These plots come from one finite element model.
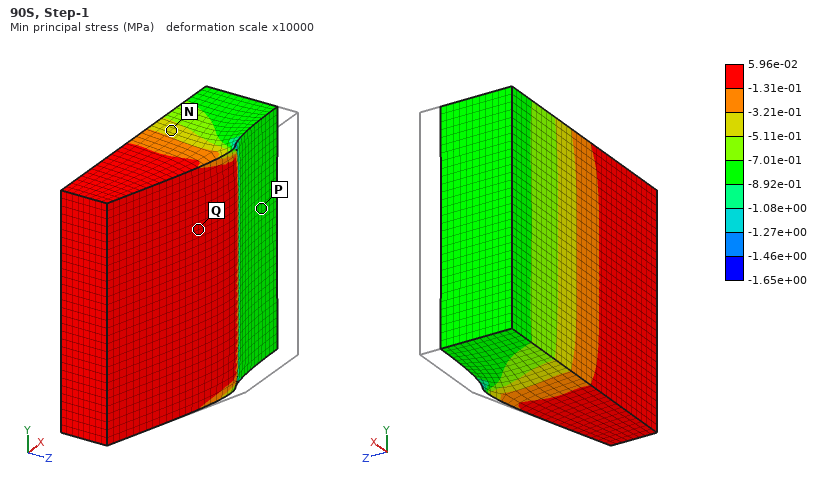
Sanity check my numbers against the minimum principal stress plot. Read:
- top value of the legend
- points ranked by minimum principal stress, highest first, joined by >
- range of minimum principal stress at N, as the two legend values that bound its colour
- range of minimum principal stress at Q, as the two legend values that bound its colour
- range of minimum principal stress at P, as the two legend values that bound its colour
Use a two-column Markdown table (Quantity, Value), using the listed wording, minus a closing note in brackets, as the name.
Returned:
| Quantity | Value |
|---|---|
| top value of the legend | 5.96e-02 MPa |
| points ranked by minimum principal stress, highest first, joined by > | Q > N > P |
| range of minimum principal stress at N, as the two legend values that bound its colour | -5.11e-01 to -3.21e-01 MPa |
| range of minimum principal stress at Q, as the two legend values that bound its colour | -1.31e-01 to 5.96e-02 MPa |
| range of minimum principal stress at P, as the two legend values that bound its colour | -8.92e-01 to -7.01e-01 MPa |
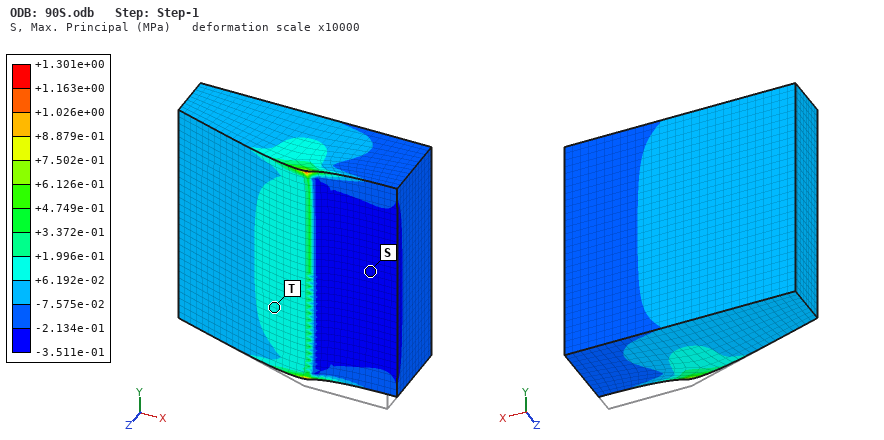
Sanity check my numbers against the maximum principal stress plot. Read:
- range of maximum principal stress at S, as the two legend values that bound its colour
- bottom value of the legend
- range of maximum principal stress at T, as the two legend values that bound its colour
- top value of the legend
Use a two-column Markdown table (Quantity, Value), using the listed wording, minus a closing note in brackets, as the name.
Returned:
| Quantity | Value |
|---|---|
| range of maximum principal stress at S, as the two legend values that bound its colour | -3.511e-01 to -2.134e-01 MPa |
| bottom value of the legend | -3.511e-01 MPa |
| range of maximum principal stress at T, as the two legend values that bound its colour | +6.192e-02 to +1.996e-01 MPa |
| top value of the legend | +1.301e+00 MPa |
